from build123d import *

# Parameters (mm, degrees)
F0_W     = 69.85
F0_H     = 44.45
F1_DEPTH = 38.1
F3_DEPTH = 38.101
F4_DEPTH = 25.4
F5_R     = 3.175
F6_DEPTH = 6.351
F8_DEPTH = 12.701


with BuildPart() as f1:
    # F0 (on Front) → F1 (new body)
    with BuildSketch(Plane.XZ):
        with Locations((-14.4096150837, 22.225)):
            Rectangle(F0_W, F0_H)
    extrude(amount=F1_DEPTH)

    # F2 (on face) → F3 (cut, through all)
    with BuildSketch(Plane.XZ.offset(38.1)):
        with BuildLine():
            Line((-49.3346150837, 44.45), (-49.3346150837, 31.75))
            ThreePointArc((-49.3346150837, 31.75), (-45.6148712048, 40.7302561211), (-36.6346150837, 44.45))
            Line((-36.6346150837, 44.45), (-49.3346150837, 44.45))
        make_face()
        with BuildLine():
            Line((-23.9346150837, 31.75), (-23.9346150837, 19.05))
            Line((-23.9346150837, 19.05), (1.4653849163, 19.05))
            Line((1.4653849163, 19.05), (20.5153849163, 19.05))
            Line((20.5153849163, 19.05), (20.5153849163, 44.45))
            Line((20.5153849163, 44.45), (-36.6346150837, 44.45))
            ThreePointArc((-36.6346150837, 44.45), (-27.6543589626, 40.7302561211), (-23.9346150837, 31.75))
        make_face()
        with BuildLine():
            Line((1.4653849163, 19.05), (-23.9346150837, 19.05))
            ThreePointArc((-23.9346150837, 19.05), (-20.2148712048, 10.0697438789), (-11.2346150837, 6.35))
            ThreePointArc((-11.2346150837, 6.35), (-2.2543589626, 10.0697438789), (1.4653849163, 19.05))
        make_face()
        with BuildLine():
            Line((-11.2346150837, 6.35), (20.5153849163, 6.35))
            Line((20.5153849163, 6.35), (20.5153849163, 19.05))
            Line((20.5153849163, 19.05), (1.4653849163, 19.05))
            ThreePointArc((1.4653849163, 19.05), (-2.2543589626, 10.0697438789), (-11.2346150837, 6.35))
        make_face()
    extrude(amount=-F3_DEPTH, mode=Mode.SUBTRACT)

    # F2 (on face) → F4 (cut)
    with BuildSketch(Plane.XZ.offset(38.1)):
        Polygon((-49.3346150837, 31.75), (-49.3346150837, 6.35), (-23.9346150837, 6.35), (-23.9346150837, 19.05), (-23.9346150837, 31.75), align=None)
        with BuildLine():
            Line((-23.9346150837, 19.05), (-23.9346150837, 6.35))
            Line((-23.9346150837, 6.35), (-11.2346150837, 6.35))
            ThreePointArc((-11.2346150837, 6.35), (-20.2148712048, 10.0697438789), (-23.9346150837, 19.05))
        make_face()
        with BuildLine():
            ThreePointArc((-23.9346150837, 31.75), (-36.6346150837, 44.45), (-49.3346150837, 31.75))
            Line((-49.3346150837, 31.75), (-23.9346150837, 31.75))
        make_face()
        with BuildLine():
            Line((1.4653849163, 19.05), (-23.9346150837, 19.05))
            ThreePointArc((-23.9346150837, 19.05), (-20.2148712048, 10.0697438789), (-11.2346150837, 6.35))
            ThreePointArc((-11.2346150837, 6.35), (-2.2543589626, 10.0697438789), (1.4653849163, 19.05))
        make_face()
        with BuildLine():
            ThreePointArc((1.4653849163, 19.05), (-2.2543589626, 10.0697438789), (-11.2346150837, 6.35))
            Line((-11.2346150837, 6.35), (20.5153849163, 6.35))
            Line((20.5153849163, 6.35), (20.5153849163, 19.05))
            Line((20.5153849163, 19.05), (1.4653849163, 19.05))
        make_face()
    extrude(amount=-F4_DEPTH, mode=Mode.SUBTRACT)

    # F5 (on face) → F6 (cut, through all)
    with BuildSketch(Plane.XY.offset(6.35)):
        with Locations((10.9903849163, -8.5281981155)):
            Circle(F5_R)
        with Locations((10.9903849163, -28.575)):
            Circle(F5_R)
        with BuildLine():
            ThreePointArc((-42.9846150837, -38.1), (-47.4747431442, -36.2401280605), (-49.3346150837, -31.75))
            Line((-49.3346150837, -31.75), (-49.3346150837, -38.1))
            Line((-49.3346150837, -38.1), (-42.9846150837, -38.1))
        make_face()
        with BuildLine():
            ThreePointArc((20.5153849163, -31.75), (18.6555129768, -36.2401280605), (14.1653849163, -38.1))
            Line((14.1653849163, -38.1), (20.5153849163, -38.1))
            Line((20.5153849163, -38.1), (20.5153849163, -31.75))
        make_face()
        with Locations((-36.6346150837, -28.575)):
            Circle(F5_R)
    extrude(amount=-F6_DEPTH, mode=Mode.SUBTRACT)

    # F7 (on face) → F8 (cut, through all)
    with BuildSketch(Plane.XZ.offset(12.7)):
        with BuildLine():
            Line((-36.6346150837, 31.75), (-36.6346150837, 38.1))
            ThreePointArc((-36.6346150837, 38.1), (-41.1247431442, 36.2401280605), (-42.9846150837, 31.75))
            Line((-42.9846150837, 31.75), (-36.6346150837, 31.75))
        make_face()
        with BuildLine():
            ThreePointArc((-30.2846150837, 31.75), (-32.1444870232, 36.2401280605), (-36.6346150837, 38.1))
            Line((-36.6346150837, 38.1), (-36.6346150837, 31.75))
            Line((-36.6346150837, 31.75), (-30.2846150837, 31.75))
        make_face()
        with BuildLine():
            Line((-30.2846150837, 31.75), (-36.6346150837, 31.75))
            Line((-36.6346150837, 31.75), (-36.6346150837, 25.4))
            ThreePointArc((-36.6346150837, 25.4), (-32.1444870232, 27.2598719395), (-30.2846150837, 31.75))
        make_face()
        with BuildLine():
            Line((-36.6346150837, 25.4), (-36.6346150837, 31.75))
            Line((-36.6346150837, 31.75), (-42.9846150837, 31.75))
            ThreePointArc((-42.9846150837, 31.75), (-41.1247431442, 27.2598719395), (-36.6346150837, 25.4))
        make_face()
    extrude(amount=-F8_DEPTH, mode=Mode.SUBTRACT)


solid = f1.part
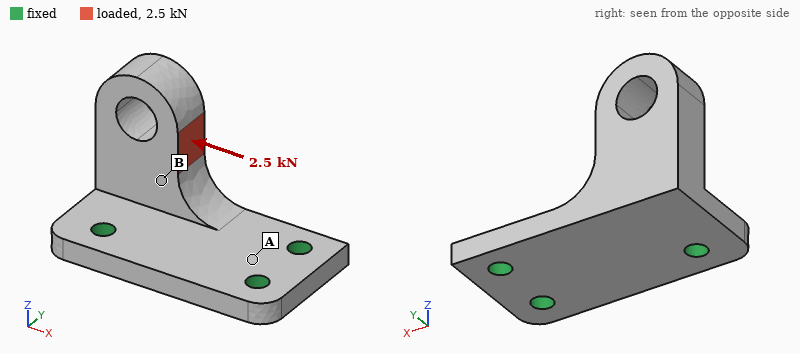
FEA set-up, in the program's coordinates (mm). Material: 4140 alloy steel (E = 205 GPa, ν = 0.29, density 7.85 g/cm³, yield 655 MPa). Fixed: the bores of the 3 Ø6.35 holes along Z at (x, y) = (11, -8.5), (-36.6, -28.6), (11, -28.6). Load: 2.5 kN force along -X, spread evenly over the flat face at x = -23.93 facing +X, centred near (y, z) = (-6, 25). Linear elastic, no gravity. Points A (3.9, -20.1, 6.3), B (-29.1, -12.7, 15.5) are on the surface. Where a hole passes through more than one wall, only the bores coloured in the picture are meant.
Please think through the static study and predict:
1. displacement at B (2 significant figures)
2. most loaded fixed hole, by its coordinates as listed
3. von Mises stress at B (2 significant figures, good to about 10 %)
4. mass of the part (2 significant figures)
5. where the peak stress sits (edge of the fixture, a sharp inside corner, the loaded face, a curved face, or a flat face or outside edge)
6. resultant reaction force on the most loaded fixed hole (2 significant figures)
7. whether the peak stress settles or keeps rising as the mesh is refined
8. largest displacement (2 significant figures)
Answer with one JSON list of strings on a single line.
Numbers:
["22 µm", "(-36.6, -28.6)", "34 MPa", "210 g", "edge of the fixture", "1.5 kN", "keeps rising", "78 µm"]
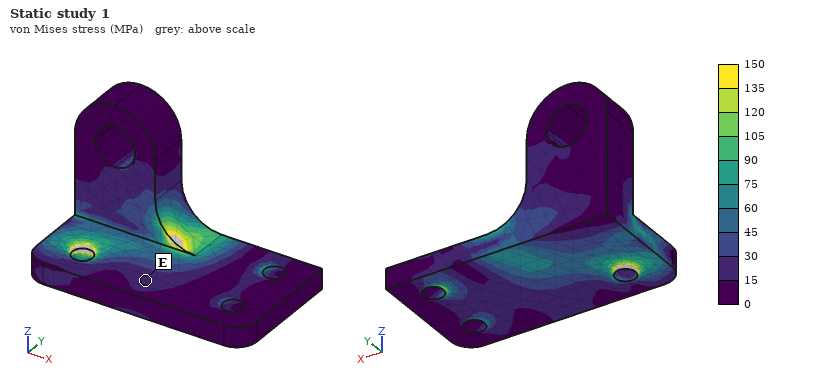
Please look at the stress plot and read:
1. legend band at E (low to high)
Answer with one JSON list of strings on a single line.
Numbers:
["15 to 30 MPa"]
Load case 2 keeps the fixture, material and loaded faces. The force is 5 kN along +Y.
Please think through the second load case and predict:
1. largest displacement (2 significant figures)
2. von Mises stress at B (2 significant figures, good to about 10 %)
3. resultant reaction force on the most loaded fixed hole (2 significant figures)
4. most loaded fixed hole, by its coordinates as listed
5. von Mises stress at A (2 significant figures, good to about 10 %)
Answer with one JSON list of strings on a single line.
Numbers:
["0.41 mm", "140 MPa", "3.5 kN", "(-36.6, -28.6)", "100 MPa"]
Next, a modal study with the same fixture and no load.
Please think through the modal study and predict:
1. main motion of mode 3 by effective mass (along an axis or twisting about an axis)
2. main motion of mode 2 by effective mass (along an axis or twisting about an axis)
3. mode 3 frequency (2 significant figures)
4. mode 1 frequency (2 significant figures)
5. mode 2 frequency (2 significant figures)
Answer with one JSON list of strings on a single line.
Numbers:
["along Z", "along X", "7400 Hz", "2300 Hz", "4500 Hz"]
